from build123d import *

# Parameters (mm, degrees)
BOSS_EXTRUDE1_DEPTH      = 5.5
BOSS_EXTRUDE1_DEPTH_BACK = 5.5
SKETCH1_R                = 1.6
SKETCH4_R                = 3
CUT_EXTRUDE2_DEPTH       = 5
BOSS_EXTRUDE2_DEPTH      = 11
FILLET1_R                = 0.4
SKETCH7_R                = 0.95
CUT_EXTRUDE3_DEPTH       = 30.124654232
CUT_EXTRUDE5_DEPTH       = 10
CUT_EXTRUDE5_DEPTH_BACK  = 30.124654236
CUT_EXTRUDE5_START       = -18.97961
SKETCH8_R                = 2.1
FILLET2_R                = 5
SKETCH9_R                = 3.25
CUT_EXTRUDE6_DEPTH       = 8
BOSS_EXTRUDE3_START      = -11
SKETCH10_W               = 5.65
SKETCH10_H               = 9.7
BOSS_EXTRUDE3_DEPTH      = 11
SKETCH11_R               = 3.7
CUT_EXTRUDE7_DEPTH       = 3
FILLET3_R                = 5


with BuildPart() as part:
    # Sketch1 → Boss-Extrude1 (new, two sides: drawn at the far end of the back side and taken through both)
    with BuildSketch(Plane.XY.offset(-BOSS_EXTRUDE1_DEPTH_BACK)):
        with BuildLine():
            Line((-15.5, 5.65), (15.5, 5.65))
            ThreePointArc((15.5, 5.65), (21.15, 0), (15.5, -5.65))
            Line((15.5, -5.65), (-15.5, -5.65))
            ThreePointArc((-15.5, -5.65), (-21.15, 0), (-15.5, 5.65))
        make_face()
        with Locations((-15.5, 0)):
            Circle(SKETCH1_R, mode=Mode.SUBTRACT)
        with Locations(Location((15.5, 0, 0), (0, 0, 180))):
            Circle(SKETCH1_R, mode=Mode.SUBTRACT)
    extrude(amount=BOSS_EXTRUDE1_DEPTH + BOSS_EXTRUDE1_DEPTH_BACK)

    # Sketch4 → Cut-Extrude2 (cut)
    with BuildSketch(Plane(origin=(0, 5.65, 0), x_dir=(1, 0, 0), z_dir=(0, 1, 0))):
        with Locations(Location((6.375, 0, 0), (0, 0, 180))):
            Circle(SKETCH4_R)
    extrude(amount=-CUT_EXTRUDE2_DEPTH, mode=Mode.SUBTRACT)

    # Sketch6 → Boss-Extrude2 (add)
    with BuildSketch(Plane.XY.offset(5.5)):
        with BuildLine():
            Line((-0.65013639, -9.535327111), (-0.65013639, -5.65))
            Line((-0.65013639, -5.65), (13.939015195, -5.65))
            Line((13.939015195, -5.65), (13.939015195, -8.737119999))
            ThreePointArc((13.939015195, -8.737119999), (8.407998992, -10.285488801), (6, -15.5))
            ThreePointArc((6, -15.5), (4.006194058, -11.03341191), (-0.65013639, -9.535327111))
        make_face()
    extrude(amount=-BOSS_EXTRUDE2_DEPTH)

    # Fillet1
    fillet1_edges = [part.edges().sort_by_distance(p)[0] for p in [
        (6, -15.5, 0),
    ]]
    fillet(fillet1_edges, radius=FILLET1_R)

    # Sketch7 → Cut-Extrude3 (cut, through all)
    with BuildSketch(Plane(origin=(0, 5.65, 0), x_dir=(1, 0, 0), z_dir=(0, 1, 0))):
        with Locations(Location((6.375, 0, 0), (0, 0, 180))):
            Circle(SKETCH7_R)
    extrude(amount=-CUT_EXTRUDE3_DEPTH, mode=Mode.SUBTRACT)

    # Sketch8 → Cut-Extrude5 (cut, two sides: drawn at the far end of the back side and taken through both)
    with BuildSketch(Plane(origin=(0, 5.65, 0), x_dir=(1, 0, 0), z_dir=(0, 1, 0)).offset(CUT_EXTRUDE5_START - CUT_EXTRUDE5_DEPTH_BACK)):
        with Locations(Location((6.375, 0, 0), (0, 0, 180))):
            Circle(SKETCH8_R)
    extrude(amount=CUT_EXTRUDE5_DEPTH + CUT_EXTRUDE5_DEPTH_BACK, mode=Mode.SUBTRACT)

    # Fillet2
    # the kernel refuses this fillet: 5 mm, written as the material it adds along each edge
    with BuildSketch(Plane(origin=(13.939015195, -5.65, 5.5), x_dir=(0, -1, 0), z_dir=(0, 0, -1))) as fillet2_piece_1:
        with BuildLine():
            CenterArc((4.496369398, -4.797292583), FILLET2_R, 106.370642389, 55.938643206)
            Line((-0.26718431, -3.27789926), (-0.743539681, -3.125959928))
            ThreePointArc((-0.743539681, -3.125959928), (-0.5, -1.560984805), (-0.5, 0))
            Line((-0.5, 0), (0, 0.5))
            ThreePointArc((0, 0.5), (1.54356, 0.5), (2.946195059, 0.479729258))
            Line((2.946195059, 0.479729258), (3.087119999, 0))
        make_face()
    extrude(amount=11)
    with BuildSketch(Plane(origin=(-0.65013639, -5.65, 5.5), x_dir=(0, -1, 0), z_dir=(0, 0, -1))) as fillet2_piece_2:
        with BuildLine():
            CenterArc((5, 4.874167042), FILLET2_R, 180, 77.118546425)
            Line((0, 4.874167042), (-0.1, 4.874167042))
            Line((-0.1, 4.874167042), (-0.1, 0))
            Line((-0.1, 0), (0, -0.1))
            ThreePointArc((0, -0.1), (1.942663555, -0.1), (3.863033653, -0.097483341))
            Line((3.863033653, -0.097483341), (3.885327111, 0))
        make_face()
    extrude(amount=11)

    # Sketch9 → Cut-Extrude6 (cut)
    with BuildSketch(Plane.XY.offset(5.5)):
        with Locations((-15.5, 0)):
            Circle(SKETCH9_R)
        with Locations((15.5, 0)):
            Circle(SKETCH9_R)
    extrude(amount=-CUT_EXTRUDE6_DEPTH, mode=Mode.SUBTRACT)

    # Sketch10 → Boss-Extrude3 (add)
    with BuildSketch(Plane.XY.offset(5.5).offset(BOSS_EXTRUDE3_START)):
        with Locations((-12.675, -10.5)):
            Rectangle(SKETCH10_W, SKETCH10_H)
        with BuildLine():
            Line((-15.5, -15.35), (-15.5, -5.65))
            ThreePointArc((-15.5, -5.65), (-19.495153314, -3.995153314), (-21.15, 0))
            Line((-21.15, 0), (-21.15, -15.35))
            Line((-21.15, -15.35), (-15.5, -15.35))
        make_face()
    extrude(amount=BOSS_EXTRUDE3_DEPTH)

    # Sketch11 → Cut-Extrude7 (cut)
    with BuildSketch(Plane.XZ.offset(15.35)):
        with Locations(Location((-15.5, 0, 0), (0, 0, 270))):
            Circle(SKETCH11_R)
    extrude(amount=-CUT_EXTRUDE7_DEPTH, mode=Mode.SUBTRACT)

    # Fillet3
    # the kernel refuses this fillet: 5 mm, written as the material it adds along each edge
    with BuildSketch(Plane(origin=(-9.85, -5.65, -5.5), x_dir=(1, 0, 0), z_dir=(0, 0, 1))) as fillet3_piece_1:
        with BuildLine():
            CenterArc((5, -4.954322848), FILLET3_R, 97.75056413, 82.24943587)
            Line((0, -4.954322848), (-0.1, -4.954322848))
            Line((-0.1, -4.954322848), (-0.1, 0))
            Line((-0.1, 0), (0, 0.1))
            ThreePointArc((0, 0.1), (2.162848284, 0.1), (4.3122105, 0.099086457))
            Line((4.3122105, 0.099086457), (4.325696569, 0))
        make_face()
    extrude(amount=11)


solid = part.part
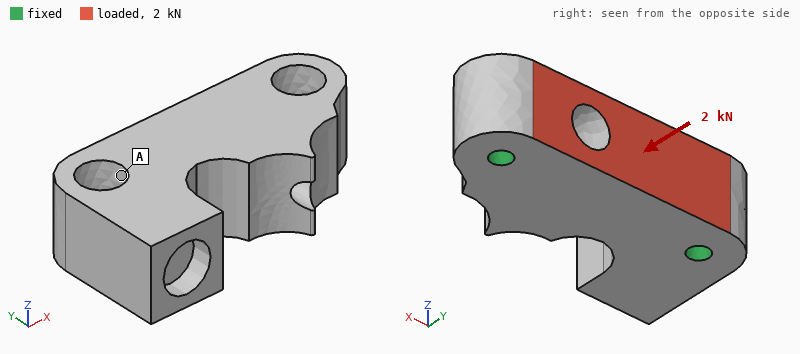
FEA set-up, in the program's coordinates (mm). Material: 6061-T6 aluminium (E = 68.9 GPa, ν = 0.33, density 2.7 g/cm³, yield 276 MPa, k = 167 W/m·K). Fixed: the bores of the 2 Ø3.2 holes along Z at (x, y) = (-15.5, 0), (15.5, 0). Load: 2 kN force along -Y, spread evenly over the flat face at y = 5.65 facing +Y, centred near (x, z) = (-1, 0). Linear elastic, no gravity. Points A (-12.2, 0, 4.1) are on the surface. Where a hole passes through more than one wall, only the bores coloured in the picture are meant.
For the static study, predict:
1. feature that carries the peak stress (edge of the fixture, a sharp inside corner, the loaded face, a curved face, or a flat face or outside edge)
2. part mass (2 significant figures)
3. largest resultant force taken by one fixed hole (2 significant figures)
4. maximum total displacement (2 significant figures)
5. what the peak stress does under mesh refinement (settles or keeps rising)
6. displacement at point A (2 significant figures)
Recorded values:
edge of the fixture
17 g
1.0 kN
47 µm
keeps rising
24 µm
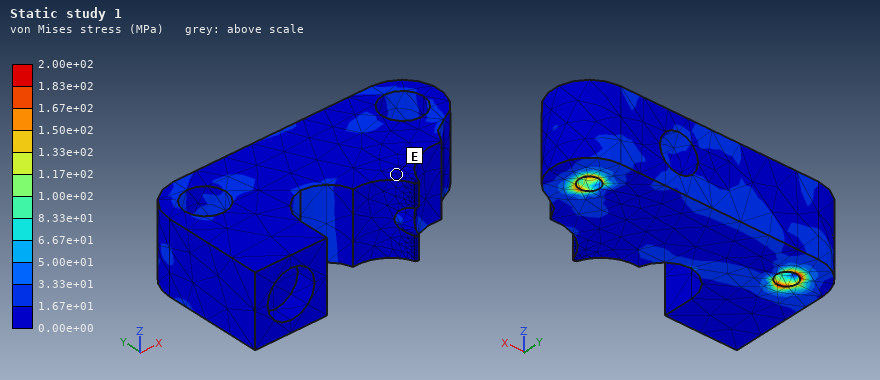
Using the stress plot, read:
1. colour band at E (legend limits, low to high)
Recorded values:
0.00e+00 to 1.67e+01 MPa
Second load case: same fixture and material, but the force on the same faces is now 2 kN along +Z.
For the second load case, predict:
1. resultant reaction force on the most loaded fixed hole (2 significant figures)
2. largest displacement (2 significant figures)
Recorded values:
1.2 kN
55 µm
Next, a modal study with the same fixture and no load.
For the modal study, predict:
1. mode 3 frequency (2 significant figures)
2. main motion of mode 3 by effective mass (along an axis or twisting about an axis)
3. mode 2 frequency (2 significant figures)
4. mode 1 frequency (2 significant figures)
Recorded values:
21 kHz
along Z
19 kHz
9000 Hz
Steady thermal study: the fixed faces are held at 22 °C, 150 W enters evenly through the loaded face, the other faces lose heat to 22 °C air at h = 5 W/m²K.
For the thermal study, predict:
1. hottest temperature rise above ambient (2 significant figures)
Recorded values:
66 K
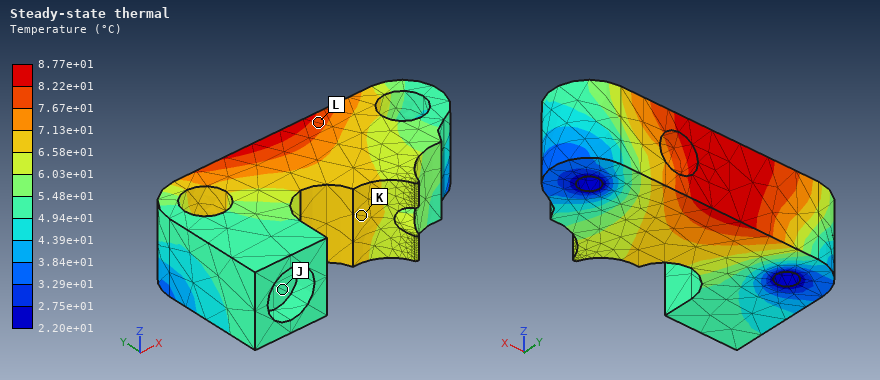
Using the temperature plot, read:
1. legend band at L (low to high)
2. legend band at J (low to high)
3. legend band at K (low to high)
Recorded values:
7.67e+01 to 8.22e+01 °C
4.94e+01 to 5.48e+01 °C
6.58e+01 to 7.13e+01 °C
